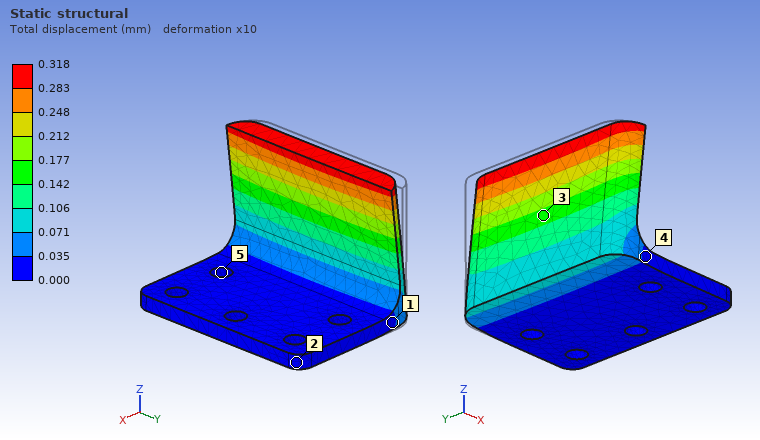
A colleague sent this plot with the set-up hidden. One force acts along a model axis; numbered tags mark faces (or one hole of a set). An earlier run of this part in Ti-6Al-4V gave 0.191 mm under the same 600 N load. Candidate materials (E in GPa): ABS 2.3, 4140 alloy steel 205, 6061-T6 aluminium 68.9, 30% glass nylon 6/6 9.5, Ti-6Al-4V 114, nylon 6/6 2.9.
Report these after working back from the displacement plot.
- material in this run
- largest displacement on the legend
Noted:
6061-T6 aluminium
0.318 mm
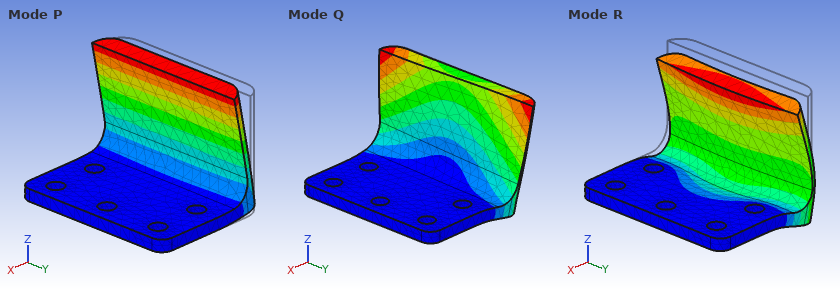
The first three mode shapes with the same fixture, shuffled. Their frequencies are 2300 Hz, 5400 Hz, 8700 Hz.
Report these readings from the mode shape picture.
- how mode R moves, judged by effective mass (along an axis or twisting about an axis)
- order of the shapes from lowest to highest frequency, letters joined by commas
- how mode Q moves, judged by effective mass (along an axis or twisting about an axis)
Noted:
along Z
P, Q, R
along Y
